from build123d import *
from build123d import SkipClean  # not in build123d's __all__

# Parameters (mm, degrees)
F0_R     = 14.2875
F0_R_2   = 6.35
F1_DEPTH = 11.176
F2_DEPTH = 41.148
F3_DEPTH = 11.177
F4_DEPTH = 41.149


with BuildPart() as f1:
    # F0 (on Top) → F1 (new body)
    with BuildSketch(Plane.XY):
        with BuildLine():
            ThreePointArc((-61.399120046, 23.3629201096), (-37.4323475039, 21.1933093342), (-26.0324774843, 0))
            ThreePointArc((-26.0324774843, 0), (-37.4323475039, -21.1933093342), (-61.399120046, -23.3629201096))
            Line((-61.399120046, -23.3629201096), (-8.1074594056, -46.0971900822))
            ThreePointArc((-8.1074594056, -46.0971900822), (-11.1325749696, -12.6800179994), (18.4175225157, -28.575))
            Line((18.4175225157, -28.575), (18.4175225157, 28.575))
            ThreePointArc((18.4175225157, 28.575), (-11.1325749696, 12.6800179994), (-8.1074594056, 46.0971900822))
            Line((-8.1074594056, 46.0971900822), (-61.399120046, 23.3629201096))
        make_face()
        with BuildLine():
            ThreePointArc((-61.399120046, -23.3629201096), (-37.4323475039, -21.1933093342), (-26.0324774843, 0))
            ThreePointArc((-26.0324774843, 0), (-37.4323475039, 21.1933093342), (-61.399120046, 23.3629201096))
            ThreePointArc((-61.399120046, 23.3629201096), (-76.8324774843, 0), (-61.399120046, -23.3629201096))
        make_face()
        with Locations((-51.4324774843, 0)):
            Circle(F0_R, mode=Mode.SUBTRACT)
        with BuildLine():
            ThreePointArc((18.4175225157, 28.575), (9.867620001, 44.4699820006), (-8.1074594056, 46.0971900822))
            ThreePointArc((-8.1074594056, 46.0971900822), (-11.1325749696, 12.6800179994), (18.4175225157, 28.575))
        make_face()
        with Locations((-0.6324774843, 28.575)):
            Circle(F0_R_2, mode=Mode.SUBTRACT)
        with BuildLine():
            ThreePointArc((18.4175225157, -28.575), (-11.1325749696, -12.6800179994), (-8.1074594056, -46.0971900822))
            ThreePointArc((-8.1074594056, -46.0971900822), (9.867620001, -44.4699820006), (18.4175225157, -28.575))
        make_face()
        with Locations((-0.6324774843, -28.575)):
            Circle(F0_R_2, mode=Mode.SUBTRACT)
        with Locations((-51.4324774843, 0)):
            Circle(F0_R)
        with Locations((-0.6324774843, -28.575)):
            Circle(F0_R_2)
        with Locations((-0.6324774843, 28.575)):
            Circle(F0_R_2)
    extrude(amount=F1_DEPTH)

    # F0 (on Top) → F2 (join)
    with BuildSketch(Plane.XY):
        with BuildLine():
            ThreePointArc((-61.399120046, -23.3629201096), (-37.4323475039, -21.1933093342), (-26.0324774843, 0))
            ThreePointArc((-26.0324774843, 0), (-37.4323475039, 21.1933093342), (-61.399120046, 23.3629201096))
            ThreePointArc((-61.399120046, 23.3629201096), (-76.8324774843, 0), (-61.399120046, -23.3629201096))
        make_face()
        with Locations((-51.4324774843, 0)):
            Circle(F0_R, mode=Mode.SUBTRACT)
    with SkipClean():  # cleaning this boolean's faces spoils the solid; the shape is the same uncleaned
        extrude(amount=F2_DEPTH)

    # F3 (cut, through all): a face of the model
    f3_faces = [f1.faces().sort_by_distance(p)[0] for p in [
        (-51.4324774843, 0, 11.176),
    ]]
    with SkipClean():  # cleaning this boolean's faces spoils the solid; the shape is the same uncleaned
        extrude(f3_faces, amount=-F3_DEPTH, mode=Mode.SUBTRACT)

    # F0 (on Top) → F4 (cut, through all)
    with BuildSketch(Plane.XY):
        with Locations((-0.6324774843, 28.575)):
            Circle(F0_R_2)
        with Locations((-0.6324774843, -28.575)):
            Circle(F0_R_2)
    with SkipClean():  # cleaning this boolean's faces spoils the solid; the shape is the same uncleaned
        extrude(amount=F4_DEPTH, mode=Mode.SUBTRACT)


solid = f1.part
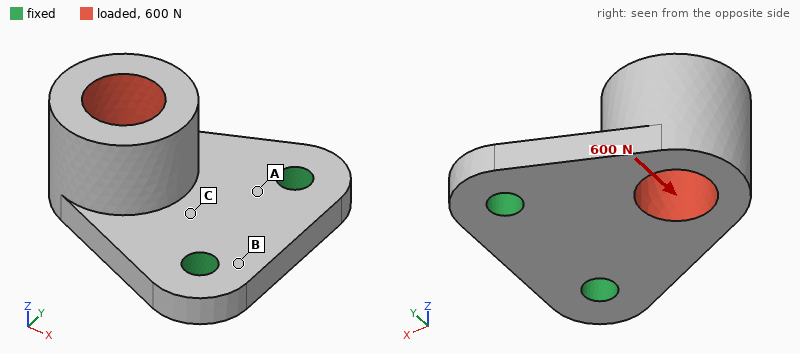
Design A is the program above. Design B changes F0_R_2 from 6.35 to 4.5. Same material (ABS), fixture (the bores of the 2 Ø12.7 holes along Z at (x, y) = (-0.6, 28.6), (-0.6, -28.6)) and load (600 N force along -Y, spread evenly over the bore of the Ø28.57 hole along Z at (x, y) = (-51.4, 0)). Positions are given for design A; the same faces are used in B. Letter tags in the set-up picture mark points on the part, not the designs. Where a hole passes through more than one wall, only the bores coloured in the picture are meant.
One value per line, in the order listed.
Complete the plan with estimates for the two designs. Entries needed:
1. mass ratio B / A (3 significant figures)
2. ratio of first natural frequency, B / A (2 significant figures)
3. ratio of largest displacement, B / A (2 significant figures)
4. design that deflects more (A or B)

1.01
0.93
1.1
B
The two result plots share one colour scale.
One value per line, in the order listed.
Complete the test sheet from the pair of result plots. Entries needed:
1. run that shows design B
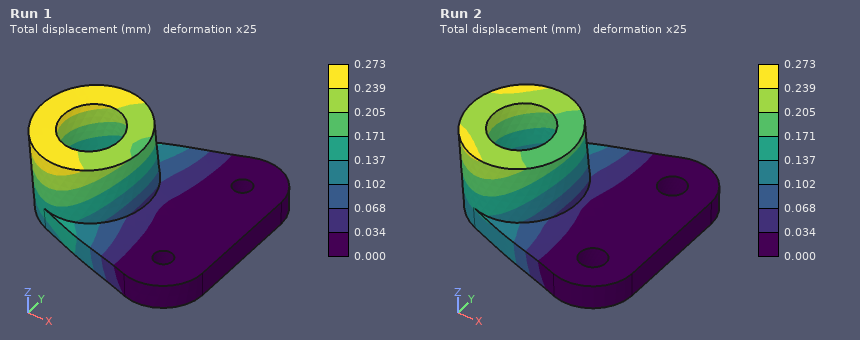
Run 1
